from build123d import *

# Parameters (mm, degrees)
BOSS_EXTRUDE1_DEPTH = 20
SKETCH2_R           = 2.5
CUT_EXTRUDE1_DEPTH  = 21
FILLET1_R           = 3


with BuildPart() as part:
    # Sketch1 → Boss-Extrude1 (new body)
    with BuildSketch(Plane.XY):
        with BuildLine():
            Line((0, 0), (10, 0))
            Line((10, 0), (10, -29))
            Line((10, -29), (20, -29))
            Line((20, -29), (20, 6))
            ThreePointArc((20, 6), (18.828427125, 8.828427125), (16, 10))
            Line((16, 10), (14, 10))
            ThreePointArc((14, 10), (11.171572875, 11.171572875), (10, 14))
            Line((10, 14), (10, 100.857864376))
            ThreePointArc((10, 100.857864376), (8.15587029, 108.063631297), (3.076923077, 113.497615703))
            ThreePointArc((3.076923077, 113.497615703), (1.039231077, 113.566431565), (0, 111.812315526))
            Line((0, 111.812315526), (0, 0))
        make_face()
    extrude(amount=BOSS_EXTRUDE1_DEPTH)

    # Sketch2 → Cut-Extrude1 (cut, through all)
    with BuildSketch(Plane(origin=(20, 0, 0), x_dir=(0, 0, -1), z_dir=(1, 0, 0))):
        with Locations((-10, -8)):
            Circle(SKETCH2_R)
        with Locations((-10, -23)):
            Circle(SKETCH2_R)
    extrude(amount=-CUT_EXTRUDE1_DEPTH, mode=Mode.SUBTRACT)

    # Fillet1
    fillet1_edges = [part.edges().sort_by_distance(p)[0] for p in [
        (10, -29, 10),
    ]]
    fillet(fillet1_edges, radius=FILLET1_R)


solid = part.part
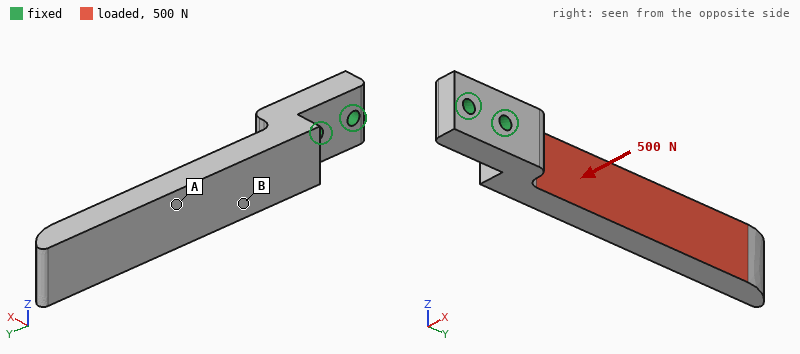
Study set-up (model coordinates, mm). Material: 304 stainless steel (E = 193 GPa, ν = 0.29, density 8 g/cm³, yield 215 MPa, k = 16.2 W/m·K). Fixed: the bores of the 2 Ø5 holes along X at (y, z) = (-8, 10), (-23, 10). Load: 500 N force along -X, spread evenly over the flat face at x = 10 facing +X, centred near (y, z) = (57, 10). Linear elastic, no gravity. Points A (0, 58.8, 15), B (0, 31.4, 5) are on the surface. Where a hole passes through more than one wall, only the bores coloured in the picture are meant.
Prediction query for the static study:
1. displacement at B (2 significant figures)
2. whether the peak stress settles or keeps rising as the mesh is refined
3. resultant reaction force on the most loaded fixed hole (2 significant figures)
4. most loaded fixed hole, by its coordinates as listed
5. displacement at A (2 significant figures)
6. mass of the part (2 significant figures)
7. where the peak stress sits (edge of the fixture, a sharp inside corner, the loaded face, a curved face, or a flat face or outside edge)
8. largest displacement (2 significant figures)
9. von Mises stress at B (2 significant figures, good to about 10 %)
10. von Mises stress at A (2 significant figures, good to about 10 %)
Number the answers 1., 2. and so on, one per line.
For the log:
1. 0.072 mm
2. keeps rising
3. 1.0 kN
4. (-8, 10)
5. 0.16 mm
6. 240 g
7. edge of the fixture
8. 0.37 mm
9. 42 MPa
10. 15 MPa
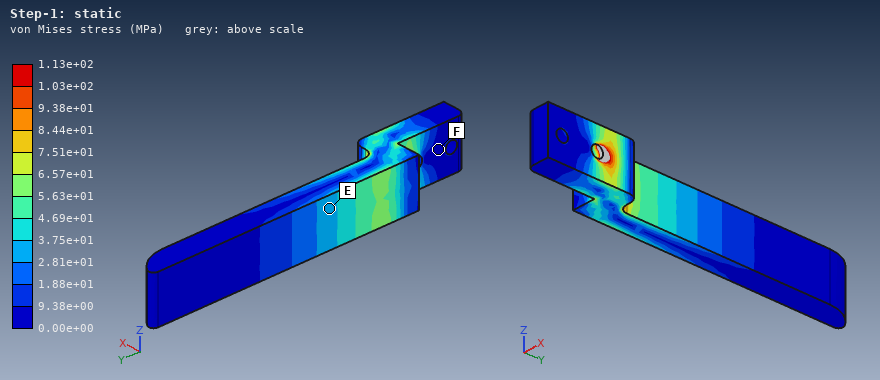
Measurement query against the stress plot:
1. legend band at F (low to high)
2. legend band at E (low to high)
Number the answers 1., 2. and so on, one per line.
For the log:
1. 0.00e+00 to 9.38e+00 MPa
2. 2.81e+01 to 3.75e+01 MPa
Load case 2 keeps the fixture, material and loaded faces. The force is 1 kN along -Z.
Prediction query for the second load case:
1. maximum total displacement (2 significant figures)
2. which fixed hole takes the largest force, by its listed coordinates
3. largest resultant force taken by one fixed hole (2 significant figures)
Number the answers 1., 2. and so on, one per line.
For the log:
1. 0.27 mm
2. (-8, 10)
3. 3.5 kN
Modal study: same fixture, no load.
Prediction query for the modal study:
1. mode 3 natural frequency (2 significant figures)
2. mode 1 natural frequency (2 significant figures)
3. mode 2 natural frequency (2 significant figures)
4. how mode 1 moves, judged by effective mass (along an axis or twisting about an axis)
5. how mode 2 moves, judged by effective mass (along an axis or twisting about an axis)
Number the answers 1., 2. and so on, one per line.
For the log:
1. 3200 Hz
2. 550 Hz
3. 910 Hz
4. along X
5. along Z
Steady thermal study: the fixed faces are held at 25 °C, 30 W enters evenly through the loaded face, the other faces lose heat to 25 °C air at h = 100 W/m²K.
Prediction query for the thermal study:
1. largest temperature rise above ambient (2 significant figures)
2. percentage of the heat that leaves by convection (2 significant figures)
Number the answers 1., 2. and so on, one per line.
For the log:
1. 74 K
2. 89 %
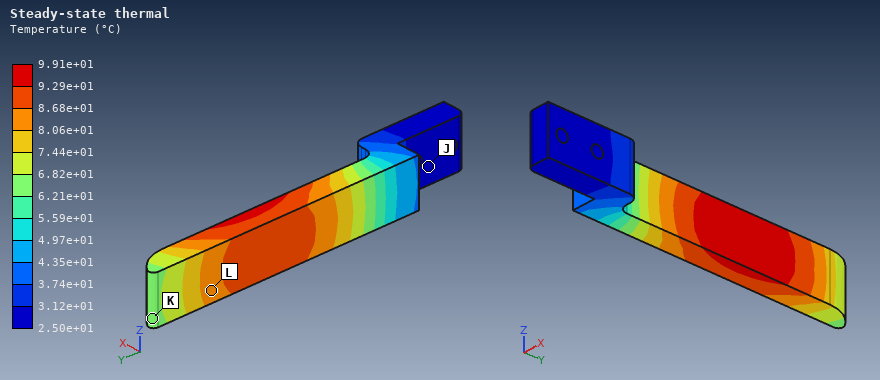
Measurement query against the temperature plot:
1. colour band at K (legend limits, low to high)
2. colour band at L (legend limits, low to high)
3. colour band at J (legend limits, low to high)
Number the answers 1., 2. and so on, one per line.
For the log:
1. 6.21e+01 to 6.82e+01 °C
2. 8.06e+01 to 8.68e+01 °C
3. 2.50e+01 to 3.12e+01 °C
